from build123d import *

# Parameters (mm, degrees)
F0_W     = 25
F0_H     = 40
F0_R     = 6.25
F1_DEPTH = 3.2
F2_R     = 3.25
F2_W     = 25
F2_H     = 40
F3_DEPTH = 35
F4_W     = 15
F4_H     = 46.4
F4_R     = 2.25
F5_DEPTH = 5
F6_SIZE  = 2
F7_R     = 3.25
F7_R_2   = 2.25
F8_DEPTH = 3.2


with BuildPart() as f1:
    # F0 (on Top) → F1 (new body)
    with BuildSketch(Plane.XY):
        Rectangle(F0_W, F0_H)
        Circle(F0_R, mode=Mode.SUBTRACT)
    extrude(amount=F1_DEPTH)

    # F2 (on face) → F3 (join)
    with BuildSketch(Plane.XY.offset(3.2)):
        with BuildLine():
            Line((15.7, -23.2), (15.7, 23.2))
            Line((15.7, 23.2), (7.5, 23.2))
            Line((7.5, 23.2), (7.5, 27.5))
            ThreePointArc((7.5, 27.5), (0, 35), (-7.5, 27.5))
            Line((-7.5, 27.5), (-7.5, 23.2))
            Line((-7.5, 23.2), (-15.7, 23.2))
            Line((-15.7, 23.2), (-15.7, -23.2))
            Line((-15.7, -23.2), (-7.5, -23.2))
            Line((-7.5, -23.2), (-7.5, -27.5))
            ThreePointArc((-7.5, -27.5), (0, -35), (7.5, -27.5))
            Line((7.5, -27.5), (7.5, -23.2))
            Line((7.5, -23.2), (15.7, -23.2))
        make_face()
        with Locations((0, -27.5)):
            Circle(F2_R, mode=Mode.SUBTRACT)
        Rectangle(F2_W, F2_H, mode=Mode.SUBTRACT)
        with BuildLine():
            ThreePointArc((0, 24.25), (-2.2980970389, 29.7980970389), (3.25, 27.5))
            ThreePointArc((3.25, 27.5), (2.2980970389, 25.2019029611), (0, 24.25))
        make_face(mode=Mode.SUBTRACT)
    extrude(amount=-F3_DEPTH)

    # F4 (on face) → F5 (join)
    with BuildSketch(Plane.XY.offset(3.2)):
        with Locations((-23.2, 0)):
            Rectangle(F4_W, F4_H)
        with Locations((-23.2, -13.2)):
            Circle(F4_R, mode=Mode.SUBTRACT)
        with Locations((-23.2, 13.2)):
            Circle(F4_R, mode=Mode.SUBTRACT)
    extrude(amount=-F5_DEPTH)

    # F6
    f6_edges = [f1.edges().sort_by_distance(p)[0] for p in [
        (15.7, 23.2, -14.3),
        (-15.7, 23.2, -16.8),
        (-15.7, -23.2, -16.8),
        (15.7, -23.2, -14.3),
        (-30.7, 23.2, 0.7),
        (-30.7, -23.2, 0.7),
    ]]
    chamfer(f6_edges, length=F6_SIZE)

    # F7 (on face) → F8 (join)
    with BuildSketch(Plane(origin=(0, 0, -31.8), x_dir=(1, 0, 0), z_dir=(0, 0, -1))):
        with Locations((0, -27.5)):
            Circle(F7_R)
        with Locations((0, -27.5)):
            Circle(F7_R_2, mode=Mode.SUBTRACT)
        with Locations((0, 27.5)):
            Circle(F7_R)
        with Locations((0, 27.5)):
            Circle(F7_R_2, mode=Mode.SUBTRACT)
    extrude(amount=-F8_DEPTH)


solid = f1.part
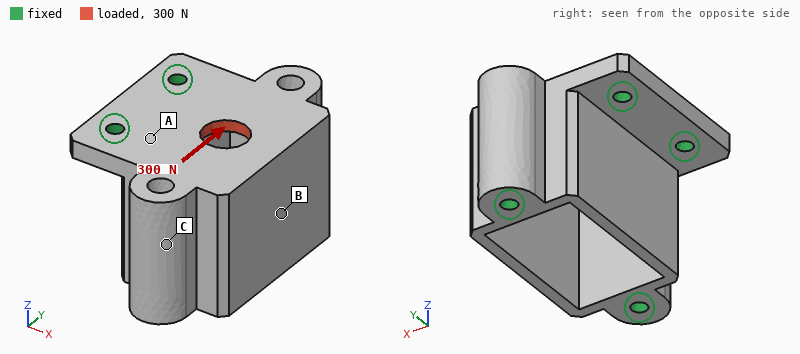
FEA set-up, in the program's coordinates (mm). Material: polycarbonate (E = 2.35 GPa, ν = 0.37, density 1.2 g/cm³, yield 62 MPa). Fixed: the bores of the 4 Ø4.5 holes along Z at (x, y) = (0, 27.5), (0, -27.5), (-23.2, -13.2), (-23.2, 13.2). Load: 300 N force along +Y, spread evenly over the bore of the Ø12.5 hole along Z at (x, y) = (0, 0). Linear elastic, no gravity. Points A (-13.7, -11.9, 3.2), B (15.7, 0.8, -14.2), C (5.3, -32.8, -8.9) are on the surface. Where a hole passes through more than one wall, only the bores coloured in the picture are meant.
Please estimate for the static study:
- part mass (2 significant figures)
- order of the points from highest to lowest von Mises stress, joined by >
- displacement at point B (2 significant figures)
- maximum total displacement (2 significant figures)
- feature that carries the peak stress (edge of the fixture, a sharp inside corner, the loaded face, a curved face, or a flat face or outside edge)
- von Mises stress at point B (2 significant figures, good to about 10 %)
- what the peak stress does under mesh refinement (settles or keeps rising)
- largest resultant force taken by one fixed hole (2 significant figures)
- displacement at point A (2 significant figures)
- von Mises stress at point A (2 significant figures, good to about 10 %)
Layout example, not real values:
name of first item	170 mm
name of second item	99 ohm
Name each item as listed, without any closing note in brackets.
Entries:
part mass	36 g
order of the points from highest to lowest von Mises stress, joined by >	A > B > C
displacement at point B	53 µm
maximum total displacement	66 µm
feature that carries the peak stress	edge of the fixture
von Mises stress at point B	1.3 MPa
what the peak stress does under mesh refinement	keeps rising
largest resultant force taken by one fixed hole	140 N
displacement at point A	16 µm
von Mises stress at point A	2.2 MPa
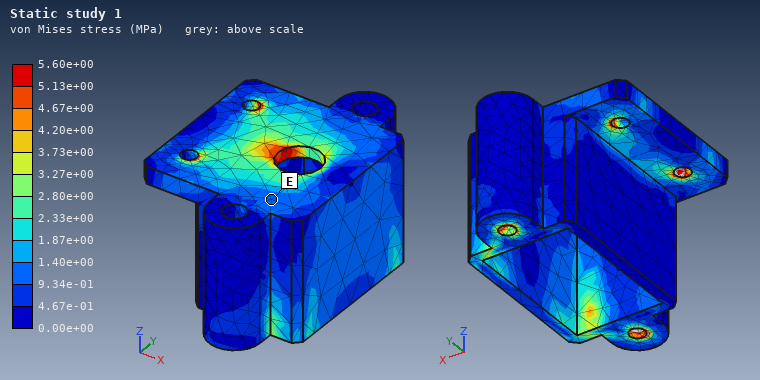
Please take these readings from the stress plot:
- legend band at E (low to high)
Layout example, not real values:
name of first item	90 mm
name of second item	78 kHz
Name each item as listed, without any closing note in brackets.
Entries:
legend band at E	9.34e-01 to 1.40e+00 MPa
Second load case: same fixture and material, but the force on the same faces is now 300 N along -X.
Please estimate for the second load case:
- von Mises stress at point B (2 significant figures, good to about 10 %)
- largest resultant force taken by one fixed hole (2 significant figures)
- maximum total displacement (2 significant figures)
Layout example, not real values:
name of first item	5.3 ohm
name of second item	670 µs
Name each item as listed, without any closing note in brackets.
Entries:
von Mises stress at point B	0.39 MPa
largest resultant force taken by one fixed hole	150 N
maximum total displacement	45 µm
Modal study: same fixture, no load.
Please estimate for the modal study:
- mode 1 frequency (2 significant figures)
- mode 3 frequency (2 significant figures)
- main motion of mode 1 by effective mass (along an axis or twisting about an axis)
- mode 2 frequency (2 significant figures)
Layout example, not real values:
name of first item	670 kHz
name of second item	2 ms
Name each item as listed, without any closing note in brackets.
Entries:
mode 1 frequency	2300 Hz
mode 3 frequency	2500 Hz
main motion of mode 1 by effective mass	along Y
mode 2 frequency	2400 Hz
